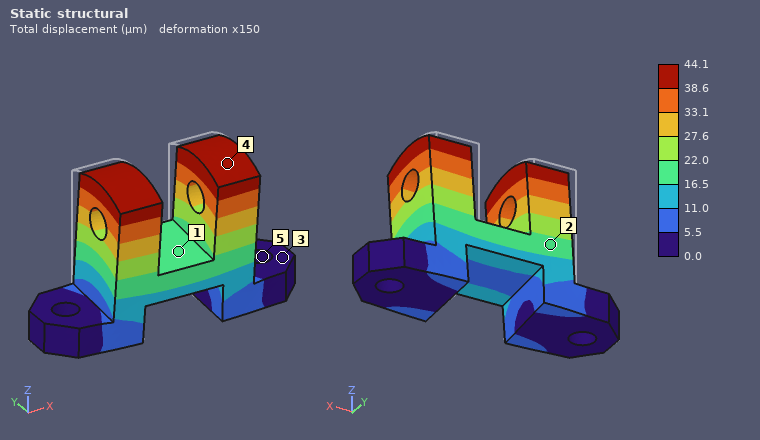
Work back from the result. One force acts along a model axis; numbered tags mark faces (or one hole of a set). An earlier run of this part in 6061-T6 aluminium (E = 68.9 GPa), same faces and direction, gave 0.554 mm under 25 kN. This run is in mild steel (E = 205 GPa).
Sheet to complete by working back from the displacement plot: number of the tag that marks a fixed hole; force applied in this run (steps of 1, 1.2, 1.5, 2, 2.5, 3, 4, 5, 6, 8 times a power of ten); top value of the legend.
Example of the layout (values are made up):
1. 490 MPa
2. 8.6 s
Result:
1. 5
2. 6 kN
3. 44.1 µm
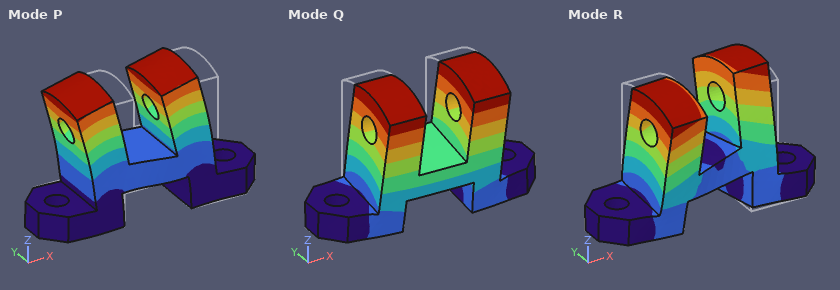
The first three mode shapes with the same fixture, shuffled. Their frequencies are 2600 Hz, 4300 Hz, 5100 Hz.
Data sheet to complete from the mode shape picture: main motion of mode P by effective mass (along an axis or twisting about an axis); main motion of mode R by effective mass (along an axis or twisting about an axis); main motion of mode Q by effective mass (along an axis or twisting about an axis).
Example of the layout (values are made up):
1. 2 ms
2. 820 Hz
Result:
1. along X
2. twisting about Z
3. along Y
